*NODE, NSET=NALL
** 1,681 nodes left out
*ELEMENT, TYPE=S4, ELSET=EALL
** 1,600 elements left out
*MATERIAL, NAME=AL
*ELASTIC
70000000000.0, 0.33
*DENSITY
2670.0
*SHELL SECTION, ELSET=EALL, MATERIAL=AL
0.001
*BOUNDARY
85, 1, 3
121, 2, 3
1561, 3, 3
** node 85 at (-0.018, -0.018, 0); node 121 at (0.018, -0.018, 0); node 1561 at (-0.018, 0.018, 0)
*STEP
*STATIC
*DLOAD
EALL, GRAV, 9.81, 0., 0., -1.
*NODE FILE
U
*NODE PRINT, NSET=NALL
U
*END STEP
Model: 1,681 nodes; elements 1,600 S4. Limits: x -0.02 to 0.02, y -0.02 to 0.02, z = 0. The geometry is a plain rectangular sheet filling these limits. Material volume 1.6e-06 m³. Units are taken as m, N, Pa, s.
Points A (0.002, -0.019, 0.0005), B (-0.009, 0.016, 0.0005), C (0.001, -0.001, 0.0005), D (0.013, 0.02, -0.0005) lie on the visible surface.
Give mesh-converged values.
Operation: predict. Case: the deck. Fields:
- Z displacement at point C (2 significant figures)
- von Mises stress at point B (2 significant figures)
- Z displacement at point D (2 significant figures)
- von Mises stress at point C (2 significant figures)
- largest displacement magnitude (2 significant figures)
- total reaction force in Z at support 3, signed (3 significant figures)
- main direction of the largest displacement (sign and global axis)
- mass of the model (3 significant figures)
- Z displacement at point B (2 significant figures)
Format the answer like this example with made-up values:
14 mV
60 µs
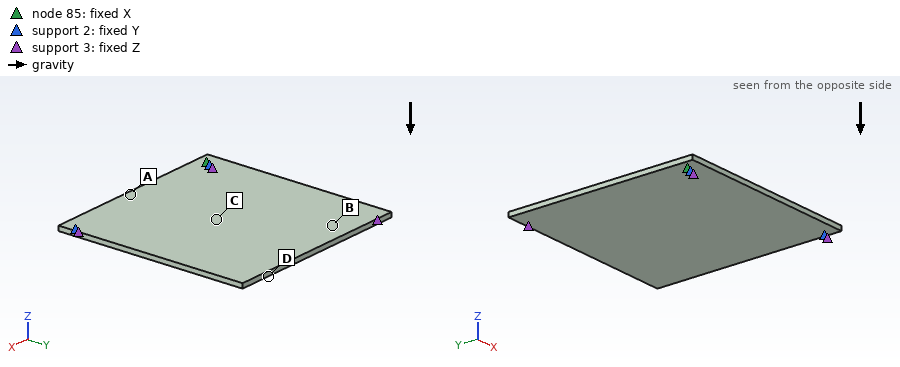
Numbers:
-4.8e-07 m
60000 Pa
-1.2e-06 m
54000 Pa
1.4e-06 m
0.0419 N
-Z
0.00427 kg
-3.9e-07 m
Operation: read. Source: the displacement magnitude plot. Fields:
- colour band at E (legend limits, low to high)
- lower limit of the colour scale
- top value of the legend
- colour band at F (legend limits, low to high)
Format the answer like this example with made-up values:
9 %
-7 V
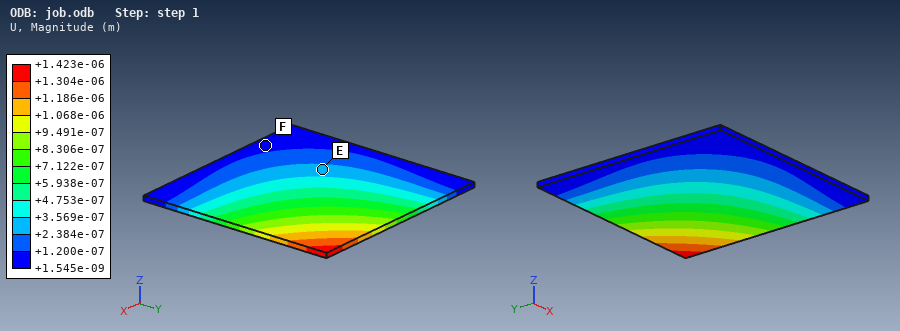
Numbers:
+2.384e-07 to +3.569e-07 m
+1.545e-09 m
+1.423e-06 m
+1.545e-09 to +1.200e-07 m
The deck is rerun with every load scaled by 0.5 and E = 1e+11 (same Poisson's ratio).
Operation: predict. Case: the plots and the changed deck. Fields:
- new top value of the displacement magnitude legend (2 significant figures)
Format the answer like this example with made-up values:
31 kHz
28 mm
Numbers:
5.0e-07 m
